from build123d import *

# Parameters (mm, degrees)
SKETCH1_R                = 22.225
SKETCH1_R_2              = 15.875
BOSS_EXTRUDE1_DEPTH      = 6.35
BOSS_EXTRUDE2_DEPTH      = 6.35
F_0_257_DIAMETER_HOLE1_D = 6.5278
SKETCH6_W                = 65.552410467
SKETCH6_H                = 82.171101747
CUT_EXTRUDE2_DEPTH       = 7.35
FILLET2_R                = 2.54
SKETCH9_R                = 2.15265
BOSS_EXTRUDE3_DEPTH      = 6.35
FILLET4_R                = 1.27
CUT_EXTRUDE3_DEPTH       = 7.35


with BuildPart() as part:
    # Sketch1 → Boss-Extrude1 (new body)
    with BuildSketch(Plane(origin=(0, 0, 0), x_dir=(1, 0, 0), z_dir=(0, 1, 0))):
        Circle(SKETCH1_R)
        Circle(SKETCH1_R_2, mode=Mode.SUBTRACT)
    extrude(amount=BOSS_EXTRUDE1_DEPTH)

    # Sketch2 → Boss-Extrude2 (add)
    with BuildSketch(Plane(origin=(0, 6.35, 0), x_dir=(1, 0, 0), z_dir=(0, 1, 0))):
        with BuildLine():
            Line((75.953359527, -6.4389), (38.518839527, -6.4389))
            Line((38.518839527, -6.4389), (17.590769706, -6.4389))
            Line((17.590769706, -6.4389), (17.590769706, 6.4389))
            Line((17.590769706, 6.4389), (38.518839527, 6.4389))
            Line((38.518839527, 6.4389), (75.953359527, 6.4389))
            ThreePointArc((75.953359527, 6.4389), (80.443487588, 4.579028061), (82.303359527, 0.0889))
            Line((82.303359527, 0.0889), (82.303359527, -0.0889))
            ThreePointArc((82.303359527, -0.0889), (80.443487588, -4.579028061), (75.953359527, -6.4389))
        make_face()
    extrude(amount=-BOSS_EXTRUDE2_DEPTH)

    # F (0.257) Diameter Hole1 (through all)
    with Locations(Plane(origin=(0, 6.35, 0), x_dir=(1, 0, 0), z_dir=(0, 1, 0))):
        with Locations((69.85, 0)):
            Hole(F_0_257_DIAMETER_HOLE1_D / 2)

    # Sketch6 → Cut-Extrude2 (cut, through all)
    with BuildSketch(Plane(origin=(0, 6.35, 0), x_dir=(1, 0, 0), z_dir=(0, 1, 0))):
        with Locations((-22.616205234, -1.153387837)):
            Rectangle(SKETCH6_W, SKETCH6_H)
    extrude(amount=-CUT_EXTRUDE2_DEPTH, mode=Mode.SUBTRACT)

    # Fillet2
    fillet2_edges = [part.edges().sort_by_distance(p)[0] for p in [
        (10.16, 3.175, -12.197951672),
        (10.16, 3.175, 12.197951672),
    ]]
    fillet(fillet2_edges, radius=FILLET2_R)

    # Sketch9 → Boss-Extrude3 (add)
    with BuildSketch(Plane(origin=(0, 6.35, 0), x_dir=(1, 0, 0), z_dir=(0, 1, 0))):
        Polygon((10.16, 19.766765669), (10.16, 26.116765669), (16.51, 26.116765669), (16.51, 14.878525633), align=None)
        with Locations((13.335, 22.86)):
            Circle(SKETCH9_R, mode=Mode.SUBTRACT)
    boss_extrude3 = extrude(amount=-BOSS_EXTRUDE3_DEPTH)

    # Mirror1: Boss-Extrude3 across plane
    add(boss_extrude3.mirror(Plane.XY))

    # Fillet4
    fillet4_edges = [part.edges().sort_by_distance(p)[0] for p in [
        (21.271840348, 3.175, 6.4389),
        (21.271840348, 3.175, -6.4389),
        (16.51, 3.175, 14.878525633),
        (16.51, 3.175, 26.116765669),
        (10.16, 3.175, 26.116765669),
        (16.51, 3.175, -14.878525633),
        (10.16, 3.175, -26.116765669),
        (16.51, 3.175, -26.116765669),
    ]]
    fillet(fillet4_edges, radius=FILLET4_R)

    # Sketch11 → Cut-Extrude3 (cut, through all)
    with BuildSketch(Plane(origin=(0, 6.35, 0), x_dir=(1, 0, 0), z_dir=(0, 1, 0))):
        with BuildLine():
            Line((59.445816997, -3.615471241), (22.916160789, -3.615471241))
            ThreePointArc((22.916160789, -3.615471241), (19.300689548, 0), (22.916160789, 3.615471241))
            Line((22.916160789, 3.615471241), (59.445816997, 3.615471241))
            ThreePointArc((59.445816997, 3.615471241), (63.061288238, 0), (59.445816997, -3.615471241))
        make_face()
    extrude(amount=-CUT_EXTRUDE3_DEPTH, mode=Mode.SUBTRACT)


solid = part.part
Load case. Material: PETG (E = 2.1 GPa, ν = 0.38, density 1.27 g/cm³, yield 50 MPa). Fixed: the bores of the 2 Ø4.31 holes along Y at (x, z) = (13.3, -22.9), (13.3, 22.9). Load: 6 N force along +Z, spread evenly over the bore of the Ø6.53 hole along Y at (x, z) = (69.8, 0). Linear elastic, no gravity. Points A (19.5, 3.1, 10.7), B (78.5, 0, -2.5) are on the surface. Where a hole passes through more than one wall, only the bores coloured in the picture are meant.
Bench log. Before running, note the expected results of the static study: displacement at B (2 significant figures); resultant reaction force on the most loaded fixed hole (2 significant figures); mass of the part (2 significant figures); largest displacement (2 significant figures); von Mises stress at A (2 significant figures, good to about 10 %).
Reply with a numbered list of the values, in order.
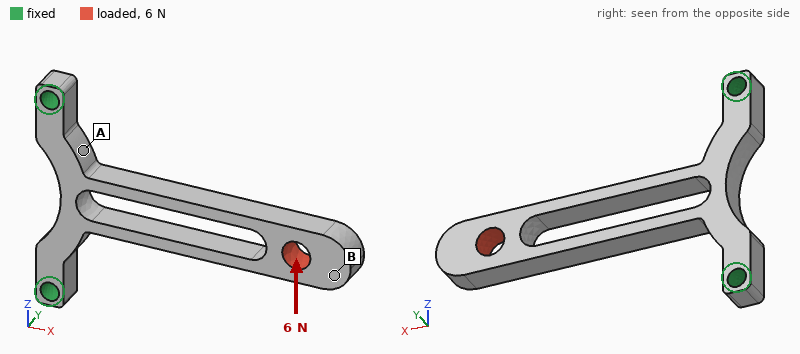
1. 0.94 mm
2. 11 N
3. 6.0 g
4. 0.96 mm
5. 1.4 MPa
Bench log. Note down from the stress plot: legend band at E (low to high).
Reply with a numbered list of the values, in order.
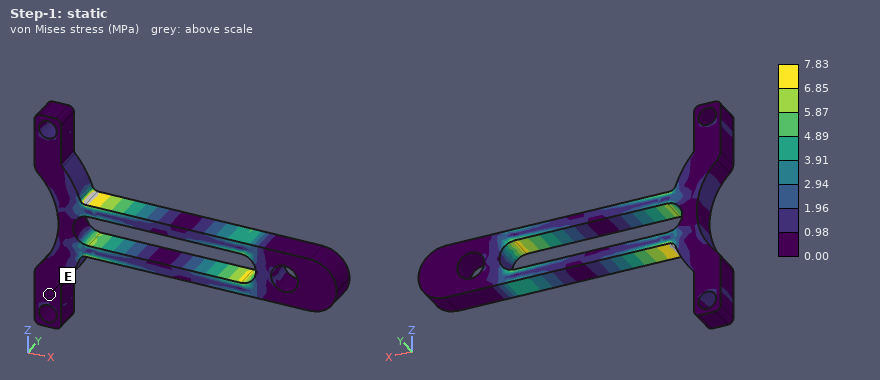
1. 0.00 to 0.98 MPa
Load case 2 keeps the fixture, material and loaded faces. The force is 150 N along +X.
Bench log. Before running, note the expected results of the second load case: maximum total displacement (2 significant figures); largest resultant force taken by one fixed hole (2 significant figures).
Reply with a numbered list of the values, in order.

1. 0.24 mm
2. 150 N
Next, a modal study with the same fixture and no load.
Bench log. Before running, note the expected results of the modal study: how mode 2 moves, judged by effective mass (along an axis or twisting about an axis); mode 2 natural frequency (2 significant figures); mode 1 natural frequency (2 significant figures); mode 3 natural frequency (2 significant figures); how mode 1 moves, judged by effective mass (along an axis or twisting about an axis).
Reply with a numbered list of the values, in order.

1. along Z
2. 270 Hz
3. 190 Hz
4. 960 Hz
5. along Y
